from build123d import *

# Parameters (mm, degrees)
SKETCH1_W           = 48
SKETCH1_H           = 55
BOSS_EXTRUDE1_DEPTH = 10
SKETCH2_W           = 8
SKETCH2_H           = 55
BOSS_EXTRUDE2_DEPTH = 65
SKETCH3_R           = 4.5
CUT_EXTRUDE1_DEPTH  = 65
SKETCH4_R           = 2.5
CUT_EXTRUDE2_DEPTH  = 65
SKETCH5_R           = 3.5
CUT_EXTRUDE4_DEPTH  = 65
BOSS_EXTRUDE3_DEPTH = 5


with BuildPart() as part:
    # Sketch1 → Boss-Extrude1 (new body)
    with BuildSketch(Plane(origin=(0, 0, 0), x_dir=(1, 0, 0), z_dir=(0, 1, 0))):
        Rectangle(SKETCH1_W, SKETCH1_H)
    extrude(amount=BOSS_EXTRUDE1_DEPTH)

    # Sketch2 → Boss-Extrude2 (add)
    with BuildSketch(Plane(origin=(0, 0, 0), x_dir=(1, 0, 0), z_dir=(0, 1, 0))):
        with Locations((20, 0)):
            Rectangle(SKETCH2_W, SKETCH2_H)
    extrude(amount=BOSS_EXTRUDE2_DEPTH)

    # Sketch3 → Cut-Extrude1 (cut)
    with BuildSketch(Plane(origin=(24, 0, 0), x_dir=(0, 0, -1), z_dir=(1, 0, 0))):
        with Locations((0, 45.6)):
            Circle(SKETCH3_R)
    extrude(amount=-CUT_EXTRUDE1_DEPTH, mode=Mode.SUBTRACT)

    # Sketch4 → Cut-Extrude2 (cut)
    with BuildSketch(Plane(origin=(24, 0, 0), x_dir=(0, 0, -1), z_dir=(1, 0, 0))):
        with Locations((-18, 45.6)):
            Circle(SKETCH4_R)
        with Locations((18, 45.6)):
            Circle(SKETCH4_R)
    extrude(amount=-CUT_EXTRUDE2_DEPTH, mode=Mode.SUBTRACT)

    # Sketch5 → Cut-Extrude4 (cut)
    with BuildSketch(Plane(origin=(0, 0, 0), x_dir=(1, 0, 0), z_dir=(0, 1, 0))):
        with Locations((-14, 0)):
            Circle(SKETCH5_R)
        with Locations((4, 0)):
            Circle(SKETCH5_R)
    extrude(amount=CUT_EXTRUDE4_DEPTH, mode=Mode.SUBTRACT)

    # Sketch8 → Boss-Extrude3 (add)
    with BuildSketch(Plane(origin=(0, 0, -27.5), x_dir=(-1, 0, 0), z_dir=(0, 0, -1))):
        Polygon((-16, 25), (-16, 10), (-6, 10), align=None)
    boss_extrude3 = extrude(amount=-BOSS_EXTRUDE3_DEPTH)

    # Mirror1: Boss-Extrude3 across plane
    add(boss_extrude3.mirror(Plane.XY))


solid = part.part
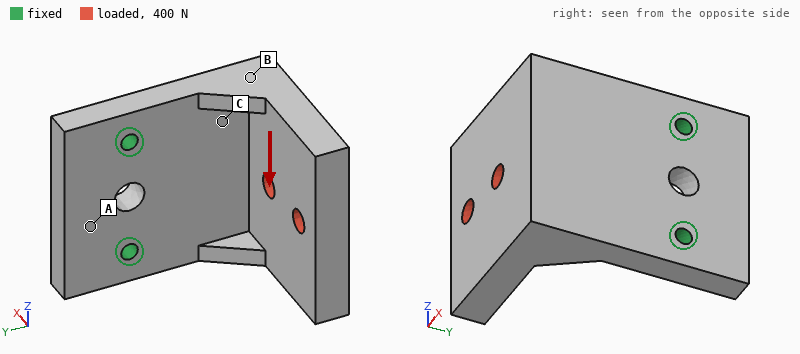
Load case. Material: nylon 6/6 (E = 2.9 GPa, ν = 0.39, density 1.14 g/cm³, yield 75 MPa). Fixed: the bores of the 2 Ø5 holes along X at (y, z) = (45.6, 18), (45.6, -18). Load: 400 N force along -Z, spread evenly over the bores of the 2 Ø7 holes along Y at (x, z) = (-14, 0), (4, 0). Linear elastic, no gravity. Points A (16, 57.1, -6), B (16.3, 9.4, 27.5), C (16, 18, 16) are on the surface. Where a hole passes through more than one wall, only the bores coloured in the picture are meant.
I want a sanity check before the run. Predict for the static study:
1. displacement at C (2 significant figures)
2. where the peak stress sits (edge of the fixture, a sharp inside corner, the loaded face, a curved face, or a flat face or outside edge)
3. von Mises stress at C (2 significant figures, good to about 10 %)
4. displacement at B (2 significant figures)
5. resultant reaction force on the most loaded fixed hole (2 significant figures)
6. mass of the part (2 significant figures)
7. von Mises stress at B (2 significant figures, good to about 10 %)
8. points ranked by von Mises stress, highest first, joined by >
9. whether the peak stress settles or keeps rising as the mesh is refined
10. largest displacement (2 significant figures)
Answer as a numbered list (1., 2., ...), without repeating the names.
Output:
1. 0.23 mm
2. edge of the fixture
3. 8.6 MPa
4. 0.48 mm
5. 520 N
6. 57 g
7. 3.7 MPa
8. C > B > A
9. keeps rising
10. 1.0 mm
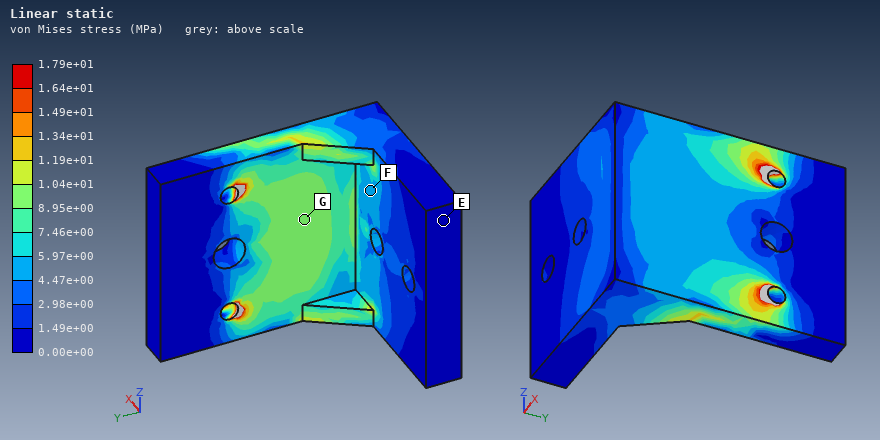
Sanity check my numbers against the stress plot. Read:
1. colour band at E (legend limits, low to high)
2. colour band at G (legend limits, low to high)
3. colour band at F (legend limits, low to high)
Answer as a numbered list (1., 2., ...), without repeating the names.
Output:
1. 0.00e+00 to 1.49e+00 MPa
2. 8.95e+00 to 1.04e+01 MPa
3. 4.47e+00 to 5.97e+00 MPa
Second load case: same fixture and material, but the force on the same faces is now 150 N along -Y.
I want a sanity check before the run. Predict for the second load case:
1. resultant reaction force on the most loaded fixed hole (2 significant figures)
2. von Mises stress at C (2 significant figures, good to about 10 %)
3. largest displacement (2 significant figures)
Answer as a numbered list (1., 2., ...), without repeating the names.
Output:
1. 76 N
2. 4.7 MPa
3. 1.1 mm
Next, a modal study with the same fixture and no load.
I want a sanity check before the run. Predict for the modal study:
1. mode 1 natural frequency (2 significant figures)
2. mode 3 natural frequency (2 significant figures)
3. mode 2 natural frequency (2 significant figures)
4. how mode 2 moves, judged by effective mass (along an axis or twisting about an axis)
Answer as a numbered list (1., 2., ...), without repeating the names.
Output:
1. 350 Hz
2. 1300 Hz
3. 700 Hz
4. along Z
